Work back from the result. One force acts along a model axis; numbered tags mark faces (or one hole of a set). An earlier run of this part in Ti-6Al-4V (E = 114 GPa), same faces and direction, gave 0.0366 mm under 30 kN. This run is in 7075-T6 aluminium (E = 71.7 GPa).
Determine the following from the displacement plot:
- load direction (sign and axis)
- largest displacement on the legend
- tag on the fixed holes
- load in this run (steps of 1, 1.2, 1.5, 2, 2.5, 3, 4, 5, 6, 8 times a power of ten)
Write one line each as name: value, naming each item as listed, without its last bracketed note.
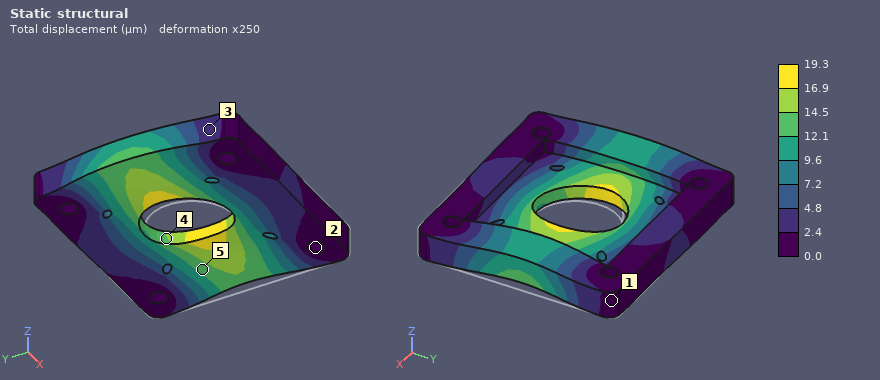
load direction: -X
largest displacement on the legend: 19.3 µm
tag on the fixed holes: 2
load in this run: 10 kN
